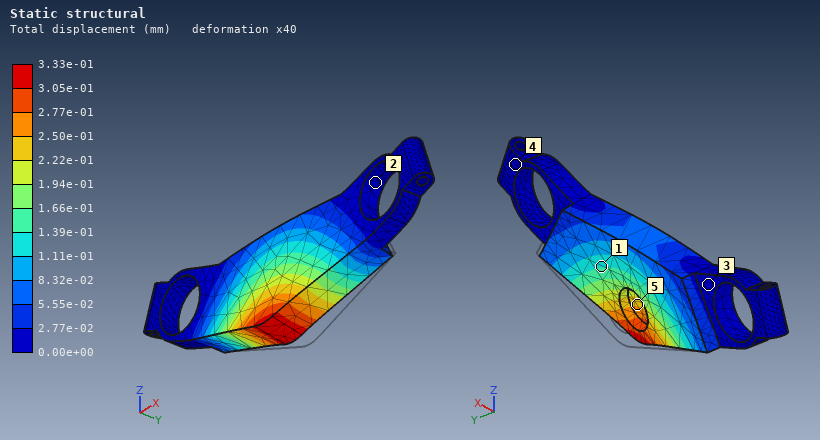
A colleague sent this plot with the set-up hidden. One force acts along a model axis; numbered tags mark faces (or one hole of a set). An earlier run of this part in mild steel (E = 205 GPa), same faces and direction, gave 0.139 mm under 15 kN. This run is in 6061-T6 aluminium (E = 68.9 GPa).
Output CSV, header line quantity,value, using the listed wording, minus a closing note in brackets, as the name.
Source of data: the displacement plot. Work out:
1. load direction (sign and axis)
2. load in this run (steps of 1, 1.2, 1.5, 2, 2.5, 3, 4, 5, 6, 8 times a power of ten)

quantity,value
load direction,-Y
load in this run,12 kN
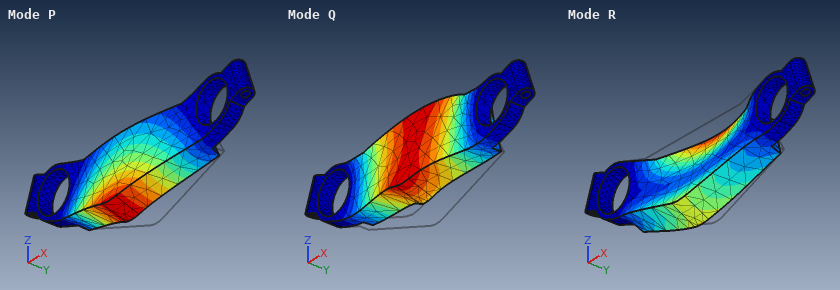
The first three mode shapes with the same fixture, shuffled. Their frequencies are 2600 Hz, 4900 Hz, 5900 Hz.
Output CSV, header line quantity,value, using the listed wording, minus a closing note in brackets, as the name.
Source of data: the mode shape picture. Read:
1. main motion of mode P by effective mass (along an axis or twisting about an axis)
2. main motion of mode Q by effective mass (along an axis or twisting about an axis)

quantity,value
main motion of mode P by effective mass,along Y
main motion of mode Q by effective mass,along Z
